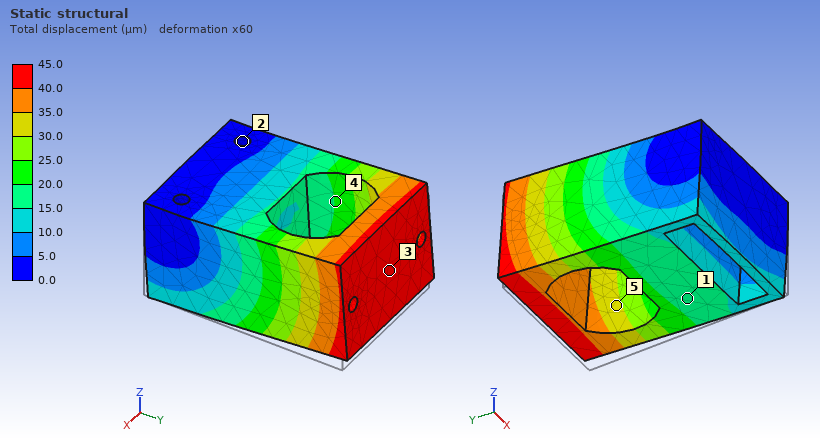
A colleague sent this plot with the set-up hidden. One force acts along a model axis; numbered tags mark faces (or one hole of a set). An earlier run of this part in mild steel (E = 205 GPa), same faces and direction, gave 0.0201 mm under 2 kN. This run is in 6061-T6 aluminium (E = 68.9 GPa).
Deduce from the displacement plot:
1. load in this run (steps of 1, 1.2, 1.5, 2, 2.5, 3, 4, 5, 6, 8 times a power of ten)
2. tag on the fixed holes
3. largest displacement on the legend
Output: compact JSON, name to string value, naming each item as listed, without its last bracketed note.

{"load in this run": "1.5 kN", "tag on the fixed holes": "2", "largest displacement on the legend": "45.0 µm"}
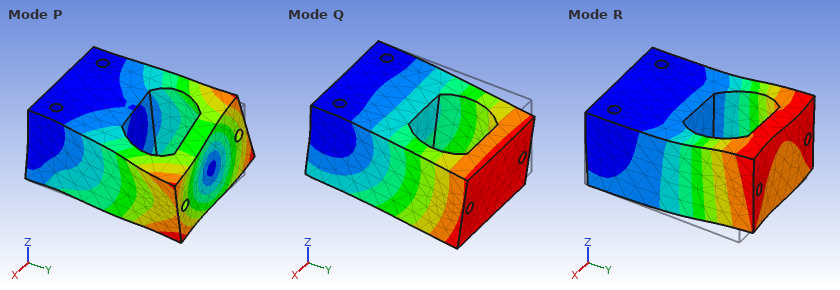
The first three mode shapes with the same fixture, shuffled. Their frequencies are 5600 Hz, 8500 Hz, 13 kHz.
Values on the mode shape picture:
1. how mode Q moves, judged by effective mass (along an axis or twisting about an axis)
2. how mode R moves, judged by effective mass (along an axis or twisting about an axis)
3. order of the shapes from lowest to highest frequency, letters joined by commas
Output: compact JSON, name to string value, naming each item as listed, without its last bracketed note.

{"how mode Q moves, judged by effective mass": "along Z", "how mode R moves, judged by effective mass": "along X", "order of the shapes from lowest to highest frequency, letters joined by commas": "Q, R, P"}
